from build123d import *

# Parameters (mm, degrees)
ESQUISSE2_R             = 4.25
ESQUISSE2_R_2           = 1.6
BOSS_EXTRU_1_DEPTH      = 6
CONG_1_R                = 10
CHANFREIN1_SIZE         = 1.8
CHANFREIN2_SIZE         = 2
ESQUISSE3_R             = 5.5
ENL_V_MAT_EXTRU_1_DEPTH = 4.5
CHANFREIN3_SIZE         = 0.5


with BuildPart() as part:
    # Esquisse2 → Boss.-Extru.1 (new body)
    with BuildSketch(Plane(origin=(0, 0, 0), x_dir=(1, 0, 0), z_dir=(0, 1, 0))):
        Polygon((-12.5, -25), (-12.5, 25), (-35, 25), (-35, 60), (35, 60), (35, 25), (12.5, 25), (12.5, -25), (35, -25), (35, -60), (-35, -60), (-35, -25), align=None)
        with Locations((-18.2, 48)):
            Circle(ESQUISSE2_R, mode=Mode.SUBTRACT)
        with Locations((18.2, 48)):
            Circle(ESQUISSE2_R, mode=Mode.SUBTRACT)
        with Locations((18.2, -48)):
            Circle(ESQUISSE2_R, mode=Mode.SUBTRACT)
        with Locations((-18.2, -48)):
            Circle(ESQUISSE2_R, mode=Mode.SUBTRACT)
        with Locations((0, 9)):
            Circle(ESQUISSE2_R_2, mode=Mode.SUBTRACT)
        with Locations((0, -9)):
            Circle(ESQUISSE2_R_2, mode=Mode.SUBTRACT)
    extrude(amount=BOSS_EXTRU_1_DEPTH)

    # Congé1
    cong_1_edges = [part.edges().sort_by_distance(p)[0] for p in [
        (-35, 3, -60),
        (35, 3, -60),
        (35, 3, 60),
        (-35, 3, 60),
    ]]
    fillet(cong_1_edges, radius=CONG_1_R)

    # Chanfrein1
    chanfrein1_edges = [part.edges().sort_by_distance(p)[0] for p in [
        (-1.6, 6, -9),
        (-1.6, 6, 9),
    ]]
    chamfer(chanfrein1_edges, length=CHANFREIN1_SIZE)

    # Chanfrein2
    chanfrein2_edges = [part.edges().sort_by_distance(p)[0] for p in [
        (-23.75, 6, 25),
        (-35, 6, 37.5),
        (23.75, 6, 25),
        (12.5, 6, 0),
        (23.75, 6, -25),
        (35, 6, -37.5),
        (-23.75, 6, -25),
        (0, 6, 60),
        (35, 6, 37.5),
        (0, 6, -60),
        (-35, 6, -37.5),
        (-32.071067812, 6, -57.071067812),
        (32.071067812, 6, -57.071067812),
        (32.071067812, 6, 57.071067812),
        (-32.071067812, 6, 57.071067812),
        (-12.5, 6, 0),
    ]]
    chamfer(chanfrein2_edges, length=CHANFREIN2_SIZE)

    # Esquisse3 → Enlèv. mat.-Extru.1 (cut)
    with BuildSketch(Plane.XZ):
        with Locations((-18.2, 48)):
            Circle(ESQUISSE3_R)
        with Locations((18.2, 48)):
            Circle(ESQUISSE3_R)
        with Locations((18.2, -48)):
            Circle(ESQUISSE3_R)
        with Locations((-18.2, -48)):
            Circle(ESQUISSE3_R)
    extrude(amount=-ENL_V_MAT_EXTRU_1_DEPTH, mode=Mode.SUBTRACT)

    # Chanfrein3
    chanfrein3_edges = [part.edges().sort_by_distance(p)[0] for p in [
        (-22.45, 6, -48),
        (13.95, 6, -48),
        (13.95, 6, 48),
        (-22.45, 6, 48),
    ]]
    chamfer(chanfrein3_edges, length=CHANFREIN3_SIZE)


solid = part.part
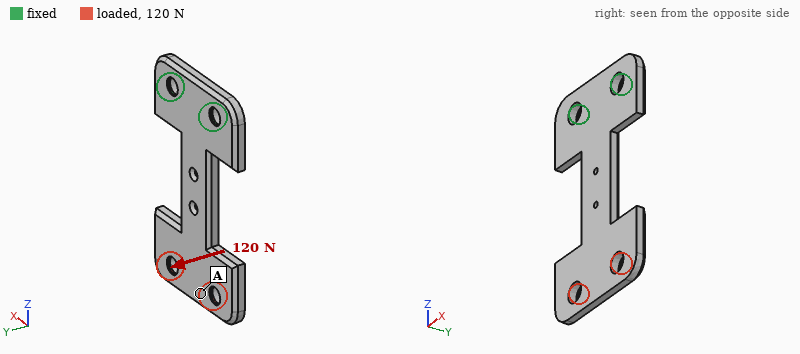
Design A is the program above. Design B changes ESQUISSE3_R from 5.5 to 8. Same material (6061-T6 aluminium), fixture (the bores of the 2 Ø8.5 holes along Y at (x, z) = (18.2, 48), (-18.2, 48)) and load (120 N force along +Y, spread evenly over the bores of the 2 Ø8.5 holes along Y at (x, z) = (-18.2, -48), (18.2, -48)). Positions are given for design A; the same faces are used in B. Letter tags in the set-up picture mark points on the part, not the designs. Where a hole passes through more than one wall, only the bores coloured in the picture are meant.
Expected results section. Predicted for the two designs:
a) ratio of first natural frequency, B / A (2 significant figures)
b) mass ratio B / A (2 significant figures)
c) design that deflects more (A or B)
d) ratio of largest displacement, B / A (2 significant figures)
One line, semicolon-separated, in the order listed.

0.93; 0.94; B; 1.2
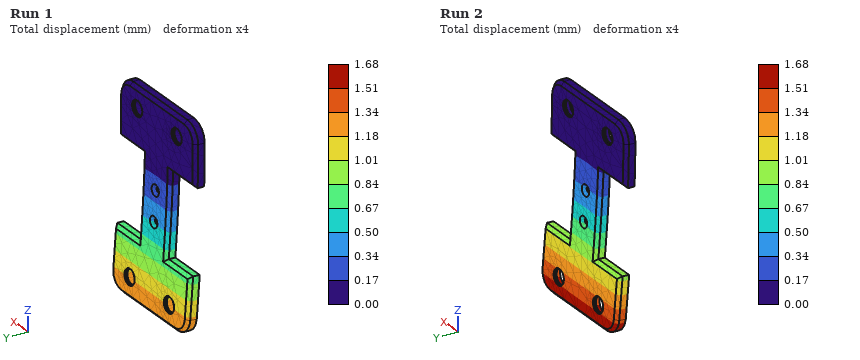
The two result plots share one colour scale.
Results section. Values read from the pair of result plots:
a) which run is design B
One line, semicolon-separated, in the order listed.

Run 2
